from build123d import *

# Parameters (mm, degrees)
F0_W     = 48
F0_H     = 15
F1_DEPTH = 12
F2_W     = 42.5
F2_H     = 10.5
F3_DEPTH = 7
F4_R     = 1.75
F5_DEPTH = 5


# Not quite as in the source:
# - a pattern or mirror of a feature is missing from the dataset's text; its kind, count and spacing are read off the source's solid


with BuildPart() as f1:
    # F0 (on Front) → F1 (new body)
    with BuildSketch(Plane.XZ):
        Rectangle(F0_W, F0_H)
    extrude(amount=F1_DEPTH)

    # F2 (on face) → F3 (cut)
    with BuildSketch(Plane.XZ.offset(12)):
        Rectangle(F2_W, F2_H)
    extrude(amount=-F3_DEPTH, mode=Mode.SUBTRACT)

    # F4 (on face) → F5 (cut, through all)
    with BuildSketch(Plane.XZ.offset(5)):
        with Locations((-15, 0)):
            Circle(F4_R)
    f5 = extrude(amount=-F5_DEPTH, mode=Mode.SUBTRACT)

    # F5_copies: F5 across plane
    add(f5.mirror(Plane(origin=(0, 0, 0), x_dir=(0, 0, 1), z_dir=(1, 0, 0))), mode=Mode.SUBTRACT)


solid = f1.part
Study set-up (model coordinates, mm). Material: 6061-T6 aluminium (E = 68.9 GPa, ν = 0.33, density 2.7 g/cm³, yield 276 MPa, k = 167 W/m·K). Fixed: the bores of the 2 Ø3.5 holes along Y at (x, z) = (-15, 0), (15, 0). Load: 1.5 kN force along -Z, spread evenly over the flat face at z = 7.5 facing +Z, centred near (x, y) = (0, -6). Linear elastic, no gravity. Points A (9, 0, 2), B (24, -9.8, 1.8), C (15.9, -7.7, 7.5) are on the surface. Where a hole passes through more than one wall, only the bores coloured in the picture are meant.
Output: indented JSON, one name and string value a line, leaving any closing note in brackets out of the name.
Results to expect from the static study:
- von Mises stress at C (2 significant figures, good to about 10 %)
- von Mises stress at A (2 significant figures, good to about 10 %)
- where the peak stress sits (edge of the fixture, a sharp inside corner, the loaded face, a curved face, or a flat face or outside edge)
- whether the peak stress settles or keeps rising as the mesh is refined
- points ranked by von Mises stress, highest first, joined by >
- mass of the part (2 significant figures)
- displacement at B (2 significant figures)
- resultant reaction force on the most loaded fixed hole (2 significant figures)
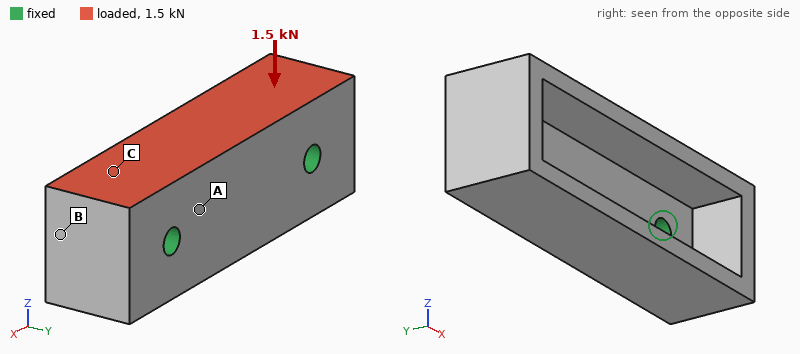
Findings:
{
  "von Mises stress at C": "28 MPa",
  "von Mises stress at A": "11 MPa",
  "where the peak stress sits": "edge of the fixture",
  "whether the peak stress settles or keeps rising as the mesh is refined": "keeps rising",
  "points ranked by von Mises stress, highest first, joined by >": "C > A > B",
  "mass of the part": "15 g",
  "displacement at B": "5.4 µm",
  "resultant reaction force on the most loaded fixed hole": "750 N"
}
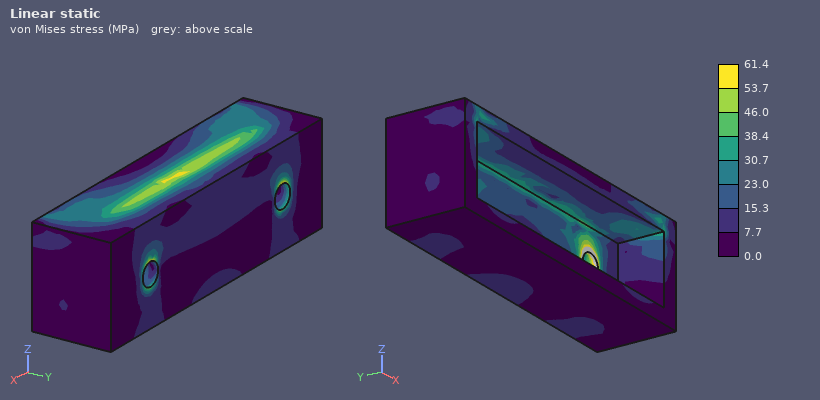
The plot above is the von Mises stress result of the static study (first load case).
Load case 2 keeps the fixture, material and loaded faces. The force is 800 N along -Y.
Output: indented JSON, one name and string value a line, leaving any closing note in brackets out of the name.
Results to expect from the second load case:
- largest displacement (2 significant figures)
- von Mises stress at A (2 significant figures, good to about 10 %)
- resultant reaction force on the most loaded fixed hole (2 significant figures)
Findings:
{
  "largest displacement": "17 µm",
  "von Mises stress at A": "12 MPa",
  "resultant reaction force on the most loaded fixed hole": "400 N"
}
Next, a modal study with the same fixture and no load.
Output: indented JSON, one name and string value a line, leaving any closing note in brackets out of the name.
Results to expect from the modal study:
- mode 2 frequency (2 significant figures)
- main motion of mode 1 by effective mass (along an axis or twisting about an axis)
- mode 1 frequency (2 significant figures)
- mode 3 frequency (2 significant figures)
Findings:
{
  "mode 2 frequency": "22 kHz",
  "main motion of mode 1 by effective mass": "along Z",
  "mode 1 frequency": "18 kHz",
  "mode 3 frequency": "24 kHz"
}
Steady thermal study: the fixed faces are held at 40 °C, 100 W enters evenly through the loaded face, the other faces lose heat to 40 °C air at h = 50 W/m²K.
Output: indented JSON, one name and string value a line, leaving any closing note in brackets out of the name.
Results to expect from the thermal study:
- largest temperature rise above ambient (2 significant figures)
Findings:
{
  "largest temperature rise above ambient": "41 K"
}
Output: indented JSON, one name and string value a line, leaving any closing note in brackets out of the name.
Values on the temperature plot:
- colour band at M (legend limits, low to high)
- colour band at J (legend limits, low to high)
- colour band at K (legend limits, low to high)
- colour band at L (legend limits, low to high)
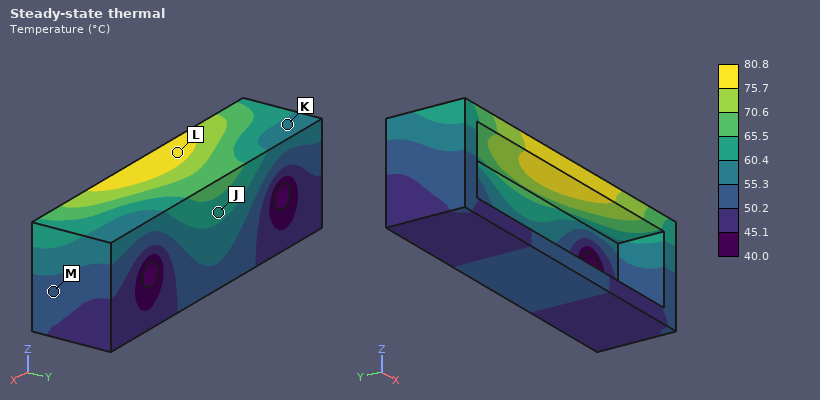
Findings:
{
  "colour band at M": "50.2 to 55.3 °C",
  "colour band at J": "60.4 to 65.5 °C",
  "colour band at K": "55.3 to 60.4 °C",
  "colour band at L": "75.7 to 80.8 °C"
}
